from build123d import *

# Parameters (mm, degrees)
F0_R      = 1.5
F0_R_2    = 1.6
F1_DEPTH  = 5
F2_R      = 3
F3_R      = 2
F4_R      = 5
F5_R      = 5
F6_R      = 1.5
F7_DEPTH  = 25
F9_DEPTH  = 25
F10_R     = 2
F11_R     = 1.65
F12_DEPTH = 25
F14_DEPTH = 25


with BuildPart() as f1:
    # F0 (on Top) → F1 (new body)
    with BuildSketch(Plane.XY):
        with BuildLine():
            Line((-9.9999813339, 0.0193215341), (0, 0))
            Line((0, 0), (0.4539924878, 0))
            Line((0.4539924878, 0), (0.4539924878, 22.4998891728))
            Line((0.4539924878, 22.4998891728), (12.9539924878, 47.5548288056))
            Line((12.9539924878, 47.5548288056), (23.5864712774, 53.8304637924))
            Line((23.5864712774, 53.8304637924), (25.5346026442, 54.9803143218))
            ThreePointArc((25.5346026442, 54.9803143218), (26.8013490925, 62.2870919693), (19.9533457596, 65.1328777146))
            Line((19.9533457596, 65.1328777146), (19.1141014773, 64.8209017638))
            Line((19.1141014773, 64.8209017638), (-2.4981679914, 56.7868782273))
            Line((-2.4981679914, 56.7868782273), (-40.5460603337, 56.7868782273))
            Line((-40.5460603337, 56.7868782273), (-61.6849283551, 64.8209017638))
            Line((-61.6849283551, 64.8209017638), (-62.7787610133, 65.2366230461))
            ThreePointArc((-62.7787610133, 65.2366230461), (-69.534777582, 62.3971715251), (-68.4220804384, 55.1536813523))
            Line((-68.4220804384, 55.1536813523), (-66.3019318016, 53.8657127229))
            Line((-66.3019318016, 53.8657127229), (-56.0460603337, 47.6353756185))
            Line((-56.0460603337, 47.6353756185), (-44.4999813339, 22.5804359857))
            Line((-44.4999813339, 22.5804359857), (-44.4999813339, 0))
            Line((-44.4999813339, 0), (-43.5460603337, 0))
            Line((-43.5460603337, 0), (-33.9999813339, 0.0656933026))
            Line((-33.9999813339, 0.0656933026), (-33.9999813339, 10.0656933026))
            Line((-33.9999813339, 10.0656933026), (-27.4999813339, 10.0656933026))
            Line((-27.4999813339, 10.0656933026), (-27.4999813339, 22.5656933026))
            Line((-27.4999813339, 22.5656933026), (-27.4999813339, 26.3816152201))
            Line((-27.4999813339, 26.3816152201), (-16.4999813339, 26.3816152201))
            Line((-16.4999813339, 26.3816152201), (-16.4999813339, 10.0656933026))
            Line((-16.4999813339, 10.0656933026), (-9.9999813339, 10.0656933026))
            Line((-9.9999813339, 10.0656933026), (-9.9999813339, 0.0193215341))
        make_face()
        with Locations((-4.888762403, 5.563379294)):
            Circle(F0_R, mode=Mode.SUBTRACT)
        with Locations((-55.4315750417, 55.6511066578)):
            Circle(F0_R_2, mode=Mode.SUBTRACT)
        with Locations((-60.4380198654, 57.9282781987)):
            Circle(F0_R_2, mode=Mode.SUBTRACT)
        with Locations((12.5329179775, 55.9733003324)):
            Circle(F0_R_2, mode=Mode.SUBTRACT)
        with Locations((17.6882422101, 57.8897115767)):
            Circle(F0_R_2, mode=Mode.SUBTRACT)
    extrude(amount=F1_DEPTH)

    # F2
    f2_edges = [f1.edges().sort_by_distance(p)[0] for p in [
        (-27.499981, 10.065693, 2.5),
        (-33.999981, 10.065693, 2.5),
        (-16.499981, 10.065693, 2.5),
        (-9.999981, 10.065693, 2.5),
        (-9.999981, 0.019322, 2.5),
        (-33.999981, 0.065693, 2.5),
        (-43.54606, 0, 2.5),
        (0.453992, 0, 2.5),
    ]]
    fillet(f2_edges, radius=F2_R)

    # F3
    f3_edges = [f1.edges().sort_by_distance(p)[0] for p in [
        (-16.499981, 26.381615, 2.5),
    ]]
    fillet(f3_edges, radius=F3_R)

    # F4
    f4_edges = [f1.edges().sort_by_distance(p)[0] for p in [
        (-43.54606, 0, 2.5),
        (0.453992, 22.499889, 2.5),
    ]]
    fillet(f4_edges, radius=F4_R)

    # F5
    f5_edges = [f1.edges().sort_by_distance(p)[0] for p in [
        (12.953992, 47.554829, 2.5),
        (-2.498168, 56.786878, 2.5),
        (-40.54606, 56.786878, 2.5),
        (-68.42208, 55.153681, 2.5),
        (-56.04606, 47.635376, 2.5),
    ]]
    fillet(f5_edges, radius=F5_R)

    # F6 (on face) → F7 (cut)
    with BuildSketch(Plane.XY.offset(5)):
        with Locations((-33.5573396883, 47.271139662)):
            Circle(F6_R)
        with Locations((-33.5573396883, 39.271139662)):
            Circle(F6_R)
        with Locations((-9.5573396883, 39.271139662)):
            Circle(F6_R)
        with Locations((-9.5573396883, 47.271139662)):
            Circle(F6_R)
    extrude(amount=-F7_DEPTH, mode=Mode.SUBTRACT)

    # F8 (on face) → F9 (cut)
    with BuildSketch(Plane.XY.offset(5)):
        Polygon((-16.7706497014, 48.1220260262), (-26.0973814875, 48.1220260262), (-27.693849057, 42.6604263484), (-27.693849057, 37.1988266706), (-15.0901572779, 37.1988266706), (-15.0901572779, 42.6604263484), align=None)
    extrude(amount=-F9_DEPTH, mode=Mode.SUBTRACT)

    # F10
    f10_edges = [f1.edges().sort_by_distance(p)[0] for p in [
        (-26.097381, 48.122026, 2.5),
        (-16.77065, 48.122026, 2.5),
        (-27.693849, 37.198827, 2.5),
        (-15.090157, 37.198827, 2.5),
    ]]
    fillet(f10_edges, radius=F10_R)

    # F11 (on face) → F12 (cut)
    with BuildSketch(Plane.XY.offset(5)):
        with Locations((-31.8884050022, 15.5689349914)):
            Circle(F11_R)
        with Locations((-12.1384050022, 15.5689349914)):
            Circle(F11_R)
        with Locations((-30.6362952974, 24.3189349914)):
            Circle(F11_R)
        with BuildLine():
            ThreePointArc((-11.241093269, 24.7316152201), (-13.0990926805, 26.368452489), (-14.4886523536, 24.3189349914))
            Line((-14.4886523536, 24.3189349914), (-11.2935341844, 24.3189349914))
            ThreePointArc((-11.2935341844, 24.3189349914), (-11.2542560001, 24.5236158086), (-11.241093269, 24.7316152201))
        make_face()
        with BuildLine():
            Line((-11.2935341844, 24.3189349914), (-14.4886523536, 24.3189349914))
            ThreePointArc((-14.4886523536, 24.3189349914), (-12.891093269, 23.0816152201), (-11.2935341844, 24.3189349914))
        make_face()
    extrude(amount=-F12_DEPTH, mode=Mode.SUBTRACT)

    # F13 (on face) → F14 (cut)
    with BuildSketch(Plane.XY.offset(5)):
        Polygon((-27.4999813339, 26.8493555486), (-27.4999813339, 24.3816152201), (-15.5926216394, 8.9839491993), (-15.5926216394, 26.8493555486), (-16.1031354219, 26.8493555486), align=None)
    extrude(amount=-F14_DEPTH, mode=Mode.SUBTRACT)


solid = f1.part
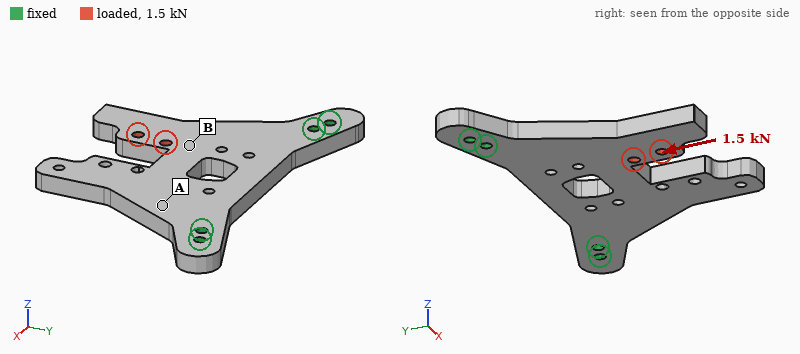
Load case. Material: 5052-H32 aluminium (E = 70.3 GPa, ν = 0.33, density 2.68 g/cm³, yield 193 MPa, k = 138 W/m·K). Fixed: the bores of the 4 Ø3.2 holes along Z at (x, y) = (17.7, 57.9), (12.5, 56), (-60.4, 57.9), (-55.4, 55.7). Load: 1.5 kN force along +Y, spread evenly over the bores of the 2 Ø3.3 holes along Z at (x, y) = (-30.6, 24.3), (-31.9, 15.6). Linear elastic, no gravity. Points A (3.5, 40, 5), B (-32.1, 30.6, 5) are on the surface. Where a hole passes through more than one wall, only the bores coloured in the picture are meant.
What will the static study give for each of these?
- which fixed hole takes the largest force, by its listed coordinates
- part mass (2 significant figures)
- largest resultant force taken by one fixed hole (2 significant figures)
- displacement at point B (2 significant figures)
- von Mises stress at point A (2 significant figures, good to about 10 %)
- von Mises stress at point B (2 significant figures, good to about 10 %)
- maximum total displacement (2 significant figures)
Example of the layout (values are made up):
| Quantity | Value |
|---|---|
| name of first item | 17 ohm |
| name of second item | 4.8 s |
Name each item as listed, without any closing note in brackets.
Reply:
| Quantity | Value |
|---|---|
| which fixed hole takes the largest force, by its listed coordinates | (-55.4, 55.7) |
| part mass | 38 g |
| largest resultant force taken by one fixed hole | 1.1 kN |
| displacement at point B | 15 µm |
| von Mises stress at point A | 7.6 MPa |
| von Mises stress at point B | 21 MPa |
| maximum total displacement | 33 µm |
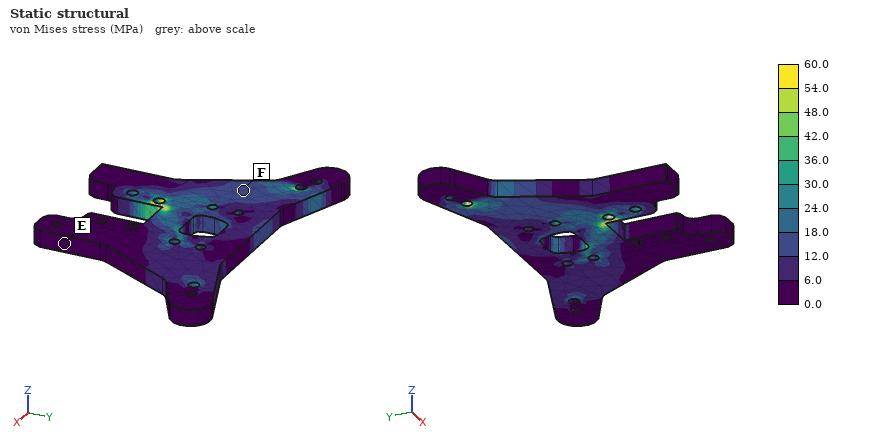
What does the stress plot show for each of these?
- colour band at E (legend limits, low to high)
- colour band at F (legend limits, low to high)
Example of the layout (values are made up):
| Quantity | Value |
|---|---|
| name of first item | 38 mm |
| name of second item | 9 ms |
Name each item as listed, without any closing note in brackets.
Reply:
| Quantity | Value |
|---|---|
| colour band at E | 0.0 to 6.0 MPa |
| colour band at F | 12.0 to 18.0 MPa |
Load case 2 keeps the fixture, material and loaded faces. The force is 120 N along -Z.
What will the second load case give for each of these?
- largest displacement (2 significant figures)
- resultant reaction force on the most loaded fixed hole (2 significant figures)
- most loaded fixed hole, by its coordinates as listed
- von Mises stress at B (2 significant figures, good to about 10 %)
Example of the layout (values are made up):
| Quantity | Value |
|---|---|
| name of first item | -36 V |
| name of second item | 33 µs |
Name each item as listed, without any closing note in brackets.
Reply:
| Quantity | Value |
|---|---|
| largest displacement | 0.21 mm |
| resultant reaction force on the most loaded fixed hole | 160 N |
| most loaded fixed hole, by its coordinates as listed | (-55.4, 55.7) |
| von Mises stress at B | 21 MPa |
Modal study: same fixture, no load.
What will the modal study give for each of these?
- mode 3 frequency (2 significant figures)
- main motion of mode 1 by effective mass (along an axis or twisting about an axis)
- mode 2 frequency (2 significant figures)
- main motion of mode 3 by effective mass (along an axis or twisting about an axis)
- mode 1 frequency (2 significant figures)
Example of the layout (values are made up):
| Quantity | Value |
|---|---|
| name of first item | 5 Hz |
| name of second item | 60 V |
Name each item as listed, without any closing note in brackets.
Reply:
| Quantity | Value |
|---|---|
| mode 3 frequency | 4900 Hz |
| main motion of mode 1 by effective mass | along Z |
| mode 2 frequency | 2600 Hz |
| main motion of mode 3 by effective mass | along Z |
| mode 1 frequency | 1300 Hz |
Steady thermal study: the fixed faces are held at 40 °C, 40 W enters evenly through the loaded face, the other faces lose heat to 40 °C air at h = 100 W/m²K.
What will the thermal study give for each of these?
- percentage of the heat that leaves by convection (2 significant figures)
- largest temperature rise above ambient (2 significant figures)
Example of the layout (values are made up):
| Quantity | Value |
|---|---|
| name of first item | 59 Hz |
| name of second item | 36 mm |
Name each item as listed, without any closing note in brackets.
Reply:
| Quantity | Value |
|---|---|
| percentage of the heat that leaves by convection | 44 % |
| largest temperature rise above ambient | 80 K |
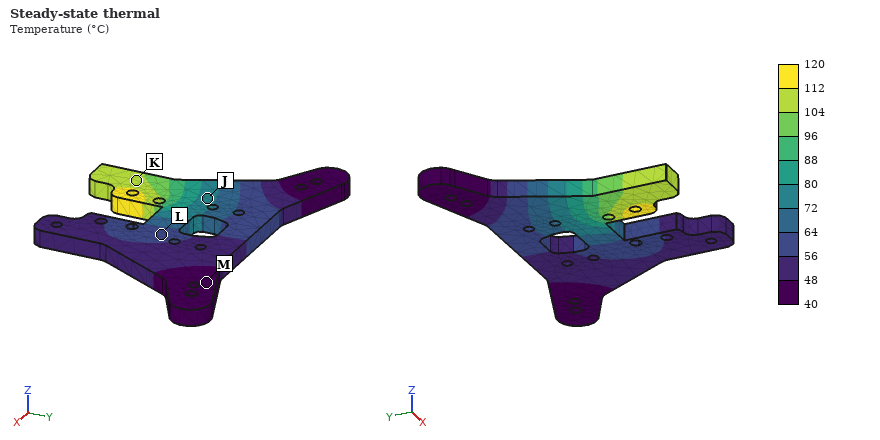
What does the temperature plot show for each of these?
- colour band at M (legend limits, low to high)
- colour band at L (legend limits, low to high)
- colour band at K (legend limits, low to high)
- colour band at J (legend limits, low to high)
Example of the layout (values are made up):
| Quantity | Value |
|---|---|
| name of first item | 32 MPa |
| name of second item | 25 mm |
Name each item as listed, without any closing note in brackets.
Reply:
| Quantity | Value |
|---|---|
| colour band at M | 40 to 48 °C |
| colour band at L | 56 to 64 °C |
| colour band at K | 104 to 112 °C |
| colour band at J | 72 to 80 °C |
